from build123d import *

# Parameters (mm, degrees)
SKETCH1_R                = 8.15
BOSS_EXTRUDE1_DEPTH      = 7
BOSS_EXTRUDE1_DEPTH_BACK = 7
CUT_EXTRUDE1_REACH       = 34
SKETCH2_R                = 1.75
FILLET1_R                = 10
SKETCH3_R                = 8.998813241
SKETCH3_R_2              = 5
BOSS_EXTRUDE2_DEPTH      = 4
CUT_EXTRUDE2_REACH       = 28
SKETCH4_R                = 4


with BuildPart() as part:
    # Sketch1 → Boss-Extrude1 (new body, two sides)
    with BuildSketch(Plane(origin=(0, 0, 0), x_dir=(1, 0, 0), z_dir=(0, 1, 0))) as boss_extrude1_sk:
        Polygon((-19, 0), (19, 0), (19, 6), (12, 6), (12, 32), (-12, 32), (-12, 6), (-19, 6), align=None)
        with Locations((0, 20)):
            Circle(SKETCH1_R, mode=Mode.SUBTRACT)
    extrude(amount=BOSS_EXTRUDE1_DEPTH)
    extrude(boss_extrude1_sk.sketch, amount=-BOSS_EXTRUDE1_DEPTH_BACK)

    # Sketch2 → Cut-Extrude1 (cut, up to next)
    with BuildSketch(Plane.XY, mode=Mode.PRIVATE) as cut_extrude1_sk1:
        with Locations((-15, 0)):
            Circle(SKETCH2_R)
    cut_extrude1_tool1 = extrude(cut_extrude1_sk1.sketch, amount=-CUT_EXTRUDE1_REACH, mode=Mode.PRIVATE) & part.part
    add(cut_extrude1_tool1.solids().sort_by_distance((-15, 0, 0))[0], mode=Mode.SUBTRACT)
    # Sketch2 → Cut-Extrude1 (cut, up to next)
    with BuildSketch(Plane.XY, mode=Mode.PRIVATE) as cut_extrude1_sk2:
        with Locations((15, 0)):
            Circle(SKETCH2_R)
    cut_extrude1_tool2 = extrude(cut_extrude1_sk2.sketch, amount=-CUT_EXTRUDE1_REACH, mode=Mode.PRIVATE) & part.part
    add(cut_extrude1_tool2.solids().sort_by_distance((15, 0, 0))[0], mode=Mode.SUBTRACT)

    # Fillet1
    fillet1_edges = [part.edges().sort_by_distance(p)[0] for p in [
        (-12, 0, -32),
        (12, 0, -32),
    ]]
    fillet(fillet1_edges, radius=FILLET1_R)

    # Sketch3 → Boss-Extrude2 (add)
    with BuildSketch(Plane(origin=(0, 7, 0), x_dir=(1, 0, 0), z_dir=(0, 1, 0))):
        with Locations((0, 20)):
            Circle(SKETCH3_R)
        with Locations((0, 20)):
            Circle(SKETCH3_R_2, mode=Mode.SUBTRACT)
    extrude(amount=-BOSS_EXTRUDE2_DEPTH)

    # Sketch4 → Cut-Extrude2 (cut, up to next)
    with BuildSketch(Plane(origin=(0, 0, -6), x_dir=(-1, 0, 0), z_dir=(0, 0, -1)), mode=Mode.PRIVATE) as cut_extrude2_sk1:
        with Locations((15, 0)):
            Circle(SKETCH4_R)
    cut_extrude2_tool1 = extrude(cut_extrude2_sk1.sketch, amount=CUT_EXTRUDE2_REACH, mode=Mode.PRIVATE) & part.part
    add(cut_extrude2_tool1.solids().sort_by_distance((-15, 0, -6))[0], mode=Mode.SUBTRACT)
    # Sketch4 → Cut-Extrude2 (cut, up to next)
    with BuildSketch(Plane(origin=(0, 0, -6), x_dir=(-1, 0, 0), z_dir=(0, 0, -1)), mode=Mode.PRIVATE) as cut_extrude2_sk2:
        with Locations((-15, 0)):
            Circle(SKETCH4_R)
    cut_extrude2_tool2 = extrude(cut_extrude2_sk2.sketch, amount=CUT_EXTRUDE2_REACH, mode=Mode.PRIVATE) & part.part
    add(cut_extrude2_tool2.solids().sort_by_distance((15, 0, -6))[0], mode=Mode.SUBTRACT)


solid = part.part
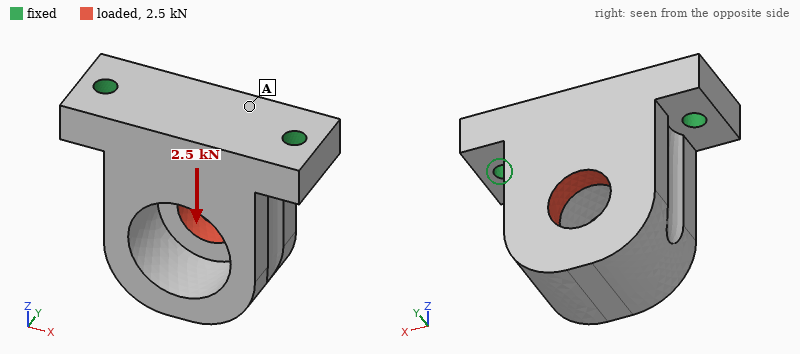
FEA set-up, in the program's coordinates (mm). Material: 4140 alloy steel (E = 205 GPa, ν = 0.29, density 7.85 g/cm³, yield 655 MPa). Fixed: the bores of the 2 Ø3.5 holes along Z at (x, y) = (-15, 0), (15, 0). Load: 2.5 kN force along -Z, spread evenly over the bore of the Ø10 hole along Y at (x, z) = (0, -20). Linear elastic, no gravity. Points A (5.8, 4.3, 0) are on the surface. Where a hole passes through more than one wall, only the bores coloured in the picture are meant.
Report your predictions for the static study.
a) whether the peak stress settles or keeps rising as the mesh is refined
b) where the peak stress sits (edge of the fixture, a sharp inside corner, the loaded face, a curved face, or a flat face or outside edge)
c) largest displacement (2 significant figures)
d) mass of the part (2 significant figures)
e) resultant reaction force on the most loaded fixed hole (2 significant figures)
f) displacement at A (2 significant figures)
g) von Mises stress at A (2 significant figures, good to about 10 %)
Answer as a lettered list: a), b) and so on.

a) keeps rising
b) edge of the fixture
c) 21 µm
d) 68 g
e) 1.3 kN
f) 4.6 µm
g) 23 MPa
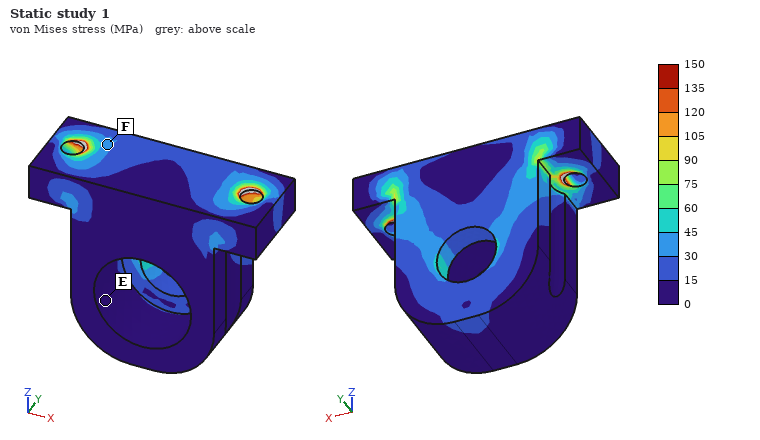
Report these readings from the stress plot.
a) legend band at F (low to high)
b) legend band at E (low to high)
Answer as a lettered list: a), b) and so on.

a) 30 to 45 MPa
b) 0 to 15 MPa
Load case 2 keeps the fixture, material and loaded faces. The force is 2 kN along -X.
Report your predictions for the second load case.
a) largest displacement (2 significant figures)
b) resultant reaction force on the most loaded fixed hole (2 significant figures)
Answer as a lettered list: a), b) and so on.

a) 11 µm
b) 1.7 kN
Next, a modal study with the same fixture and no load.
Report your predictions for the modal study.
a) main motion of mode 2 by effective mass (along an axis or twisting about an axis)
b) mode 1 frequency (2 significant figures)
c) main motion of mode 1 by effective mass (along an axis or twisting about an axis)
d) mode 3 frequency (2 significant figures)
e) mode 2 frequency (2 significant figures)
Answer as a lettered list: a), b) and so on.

a) along X
b) 6100 Hz
c) along Y
d) 20 kHz
e) 12 kHz
